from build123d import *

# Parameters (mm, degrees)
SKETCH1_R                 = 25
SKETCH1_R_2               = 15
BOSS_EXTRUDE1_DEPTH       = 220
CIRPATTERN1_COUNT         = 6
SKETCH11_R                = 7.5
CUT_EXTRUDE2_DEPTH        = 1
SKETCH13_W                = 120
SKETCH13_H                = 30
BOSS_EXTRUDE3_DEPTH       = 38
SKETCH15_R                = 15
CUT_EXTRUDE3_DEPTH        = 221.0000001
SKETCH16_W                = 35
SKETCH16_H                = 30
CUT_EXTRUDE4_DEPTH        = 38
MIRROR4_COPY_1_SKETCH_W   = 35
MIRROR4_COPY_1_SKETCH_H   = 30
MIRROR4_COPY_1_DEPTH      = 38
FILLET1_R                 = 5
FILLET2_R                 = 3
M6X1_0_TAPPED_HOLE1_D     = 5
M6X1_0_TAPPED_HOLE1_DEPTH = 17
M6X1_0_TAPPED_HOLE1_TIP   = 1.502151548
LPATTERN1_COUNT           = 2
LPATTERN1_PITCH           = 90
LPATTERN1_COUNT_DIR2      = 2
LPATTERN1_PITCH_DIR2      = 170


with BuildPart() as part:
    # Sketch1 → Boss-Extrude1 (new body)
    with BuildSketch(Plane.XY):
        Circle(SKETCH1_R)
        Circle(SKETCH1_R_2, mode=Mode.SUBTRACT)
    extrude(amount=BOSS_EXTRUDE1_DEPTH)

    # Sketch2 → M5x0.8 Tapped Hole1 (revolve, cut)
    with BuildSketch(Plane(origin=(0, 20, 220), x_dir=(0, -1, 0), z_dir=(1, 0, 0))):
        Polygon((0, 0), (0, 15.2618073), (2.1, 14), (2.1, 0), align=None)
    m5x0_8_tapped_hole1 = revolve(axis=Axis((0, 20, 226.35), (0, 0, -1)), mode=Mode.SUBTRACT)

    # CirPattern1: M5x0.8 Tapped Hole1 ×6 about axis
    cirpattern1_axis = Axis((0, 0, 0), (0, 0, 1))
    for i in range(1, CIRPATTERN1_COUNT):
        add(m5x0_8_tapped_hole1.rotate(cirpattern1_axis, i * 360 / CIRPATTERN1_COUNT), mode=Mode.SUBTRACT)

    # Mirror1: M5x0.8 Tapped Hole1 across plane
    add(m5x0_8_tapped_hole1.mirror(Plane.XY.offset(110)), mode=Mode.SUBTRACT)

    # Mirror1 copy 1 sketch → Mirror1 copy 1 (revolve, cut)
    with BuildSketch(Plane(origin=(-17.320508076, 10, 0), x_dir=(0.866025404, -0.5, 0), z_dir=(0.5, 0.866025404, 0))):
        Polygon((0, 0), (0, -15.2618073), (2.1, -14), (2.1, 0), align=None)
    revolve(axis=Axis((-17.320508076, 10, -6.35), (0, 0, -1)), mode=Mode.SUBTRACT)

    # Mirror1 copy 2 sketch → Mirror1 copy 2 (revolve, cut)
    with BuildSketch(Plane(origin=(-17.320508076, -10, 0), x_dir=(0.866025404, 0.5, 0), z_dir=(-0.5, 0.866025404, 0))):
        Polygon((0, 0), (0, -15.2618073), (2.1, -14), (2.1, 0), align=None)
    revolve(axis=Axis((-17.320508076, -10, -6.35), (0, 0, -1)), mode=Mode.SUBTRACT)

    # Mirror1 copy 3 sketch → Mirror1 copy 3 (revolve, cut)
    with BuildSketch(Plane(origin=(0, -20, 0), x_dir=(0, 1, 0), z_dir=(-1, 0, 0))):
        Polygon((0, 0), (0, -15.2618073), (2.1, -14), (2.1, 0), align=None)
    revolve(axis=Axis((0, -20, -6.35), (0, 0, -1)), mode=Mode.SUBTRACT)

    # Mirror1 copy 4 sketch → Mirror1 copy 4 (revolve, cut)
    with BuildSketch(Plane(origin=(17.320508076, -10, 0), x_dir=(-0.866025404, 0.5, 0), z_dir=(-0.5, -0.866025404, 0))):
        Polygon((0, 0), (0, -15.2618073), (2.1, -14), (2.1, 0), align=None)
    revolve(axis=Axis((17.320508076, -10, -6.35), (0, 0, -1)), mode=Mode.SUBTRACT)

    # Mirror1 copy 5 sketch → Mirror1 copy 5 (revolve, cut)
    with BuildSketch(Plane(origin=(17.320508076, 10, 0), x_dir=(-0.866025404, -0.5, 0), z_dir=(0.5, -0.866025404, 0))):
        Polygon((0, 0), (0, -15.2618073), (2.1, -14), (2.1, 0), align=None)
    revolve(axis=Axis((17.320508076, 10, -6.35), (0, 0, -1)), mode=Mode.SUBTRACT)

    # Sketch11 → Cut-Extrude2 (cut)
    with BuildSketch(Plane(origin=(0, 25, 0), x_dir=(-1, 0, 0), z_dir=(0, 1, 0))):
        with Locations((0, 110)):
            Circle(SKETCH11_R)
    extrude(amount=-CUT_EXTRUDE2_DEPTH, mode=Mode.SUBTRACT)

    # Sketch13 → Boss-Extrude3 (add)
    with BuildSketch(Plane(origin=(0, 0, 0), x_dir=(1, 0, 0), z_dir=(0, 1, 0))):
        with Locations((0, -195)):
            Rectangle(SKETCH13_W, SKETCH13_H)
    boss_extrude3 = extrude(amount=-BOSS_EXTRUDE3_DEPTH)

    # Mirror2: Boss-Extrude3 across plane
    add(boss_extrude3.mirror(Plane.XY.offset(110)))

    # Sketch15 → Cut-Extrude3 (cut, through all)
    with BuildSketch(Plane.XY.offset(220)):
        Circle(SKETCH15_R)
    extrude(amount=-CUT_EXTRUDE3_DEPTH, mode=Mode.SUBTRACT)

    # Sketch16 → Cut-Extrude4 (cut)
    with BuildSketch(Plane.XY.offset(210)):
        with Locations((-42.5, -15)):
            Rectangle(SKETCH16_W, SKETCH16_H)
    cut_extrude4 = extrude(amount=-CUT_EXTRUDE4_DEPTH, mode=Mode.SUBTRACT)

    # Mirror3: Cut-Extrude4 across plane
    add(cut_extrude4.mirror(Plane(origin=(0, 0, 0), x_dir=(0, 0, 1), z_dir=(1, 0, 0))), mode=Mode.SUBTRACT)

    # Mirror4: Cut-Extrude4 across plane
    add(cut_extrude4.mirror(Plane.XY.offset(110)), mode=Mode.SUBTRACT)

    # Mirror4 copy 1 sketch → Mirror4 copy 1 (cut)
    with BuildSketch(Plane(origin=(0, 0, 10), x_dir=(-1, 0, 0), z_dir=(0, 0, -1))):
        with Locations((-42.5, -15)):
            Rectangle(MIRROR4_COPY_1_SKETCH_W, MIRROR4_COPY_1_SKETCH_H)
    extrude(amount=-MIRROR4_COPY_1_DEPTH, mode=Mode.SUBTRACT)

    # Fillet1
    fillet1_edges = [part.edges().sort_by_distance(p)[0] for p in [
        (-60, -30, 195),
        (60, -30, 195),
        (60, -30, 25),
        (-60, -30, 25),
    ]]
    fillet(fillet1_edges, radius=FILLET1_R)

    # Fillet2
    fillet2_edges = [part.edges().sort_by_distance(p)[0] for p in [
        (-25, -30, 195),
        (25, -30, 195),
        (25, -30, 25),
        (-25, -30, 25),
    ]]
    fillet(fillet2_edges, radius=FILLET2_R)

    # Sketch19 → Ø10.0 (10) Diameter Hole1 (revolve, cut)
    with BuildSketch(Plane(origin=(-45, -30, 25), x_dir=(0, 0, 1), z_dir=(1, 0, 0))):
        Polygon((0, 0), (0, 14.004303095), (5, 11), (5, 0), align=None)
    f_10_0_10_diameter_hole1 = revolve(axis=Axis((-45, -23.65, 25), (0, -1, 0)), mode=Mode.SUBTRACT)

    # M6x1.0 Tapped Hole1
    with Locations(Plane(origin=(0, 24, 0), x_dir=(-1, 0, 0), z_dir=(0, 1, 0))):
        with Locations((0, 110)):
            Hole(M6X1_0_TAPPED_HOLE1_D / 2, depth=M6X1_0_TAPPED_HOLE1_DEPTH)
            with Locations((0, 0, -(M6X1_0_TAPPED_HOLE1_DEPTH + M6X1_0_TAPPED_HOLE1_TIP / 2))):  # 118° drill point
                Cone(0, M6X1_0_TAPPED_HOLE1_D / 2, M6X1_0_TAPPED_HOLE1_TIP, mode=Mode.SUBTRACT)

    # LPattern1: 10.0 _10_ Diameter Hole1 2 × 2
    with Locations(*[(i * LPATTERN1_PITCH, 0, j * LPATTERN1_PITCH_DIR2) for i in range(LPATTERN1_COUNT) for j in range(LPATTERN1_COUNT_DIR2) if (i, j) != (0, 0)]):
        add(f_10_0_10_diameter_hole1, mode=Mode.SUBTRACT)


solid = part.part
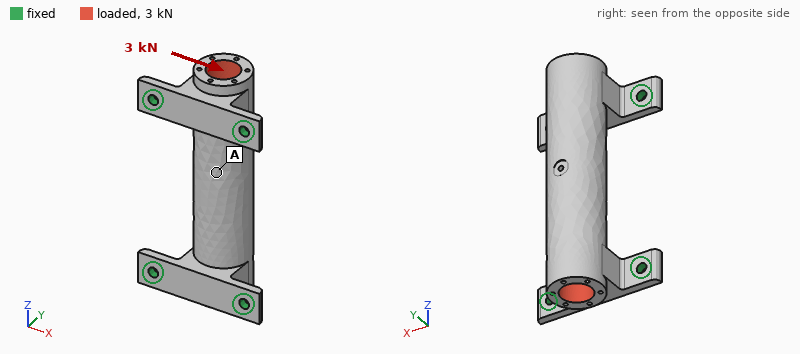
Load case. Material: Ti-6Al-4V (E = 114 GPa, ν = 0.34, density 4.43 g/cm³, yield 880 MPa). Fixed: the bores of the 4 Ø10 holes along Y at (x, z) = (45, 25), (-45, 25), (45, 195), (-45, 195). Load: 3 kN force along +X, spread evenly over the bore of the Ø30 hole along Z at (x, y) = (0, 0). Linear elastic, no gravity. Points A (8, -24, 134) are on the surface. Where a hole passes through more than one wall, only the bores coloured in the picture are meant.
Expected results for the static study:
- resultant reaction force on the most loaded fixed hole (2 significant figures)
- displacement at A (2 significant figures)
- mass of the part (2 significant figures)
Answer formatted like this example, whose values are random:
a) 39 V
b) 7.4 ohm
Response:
a) 1.1 kN
b) 6.0 µm
c) 1.6 kg
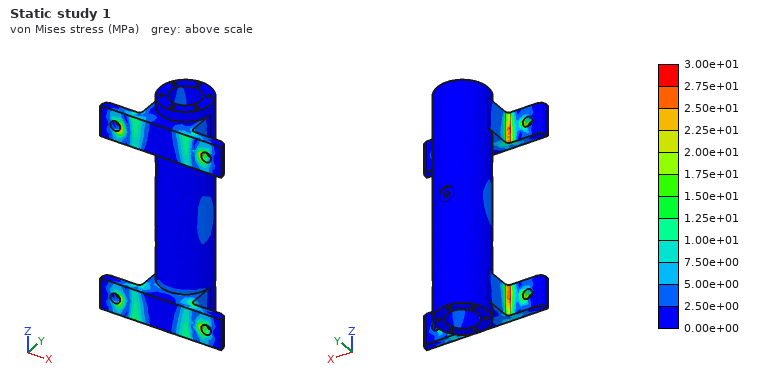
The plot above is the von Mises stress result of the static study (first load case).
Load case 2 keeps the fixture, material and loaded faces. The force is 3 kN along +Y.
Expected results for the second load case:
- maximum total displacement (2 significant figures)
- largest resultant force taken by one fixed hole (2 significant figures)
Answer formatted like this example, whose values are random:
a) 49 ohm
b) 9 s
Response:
a) 9.7 µm
b) 890 N
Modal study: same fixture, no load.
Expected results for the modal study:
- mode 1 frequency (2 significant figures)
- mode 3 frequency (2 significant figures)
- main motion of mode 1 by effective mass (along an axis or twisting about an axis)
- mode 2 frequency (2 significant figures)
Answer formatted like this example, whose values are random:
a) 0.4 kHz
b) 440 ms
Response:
a) 2300 Hz
b) 2700 Hz
c) along X
d) 2600 Hz
